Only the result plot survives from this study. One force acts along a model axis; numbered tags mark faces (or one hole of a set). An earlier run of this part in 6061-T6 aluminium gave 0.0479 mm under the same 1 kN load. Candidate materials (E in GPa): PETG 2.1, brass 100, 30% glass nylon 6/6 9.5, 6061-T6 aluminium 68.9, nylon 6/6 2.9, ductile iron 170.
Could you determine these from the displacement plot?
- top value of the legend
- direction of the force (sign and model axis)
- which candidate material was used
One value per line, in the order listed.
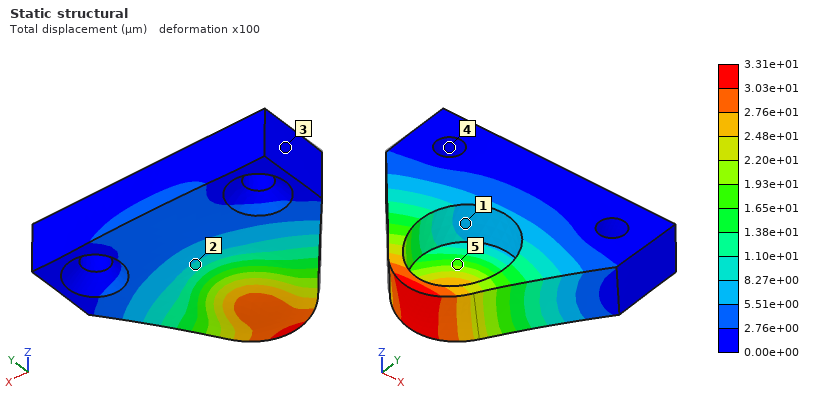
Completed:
3.31e+01 µm
-Z
brass
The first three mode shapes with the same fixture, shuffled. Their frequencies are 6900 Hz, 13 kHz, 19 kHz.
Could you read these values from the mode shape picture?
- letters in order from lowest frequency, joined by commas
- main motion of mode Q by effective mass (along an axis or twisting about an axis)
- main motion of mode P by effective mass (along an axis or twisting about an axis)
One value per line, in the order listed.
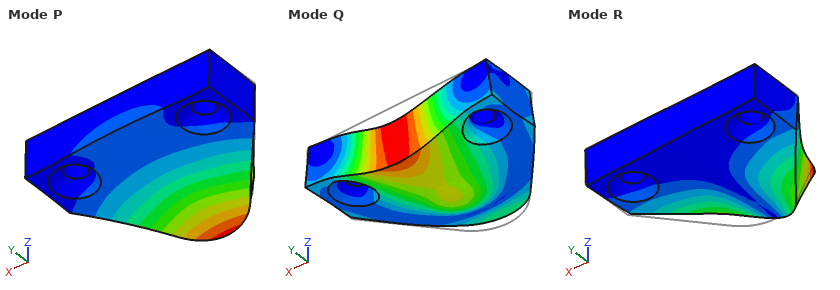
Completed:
P, R, Q
along Z
along Z
